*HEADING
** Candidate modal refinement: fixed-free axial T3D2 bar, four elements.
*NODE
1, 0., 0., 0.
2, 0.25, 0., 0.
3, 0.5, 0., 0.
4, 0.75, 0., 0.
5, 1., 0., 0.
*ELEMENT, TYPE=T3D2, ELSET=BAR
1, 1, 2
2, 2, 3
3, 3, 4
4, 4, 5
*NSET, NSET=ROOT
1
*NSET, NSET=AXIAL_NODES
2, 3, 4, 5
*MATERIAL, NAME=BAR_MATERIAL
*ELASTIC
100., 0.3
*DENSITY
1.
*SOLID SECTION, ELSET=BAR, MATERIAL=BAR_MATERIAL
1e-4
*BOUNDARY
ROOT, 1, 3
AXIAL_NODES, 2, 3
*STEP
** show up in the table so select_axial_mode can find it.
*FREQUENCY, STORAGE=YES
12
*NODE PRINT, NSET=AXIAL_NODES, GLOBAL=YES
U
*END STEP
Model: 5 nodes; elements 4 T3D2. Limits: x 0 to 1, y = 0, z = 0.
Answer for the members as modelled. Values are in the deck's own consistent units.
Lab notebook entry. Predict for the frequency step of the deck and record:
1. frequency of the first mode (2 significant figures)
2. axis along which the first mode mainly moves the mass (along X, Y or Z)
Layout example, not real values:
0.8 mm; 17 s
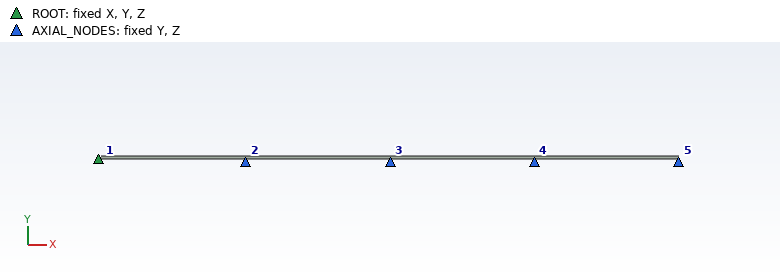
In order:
2.5 cycles per unit time; along X
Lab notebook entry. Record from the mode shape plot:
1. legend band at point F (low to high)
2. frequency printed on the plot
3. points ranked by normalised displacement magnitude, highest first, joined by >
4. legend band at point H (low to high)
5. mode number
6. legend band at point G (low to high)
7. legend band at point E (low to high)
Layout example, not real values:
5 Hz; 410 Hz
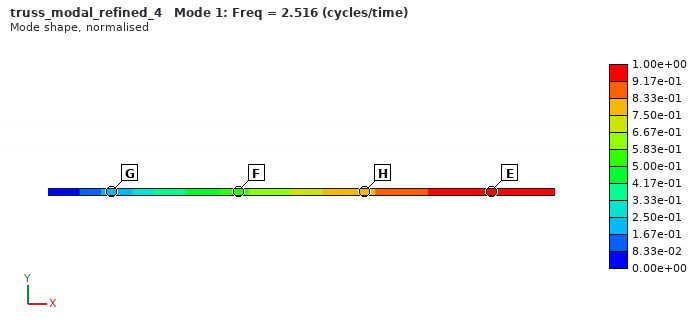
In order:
5.00e-01 to 5.83e-01; 2.516; E > H > F > G; 7.50e-01 to 8.33e-01; 1; 1.67e-01 to 2.50e-01; 9.17e-01 to 1.00e+00
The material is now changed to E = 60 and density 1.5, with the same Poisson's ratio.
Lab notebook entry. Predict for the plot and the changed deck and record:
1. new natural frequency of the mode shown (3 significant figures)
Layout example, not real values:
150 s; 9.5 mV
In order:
1.59
